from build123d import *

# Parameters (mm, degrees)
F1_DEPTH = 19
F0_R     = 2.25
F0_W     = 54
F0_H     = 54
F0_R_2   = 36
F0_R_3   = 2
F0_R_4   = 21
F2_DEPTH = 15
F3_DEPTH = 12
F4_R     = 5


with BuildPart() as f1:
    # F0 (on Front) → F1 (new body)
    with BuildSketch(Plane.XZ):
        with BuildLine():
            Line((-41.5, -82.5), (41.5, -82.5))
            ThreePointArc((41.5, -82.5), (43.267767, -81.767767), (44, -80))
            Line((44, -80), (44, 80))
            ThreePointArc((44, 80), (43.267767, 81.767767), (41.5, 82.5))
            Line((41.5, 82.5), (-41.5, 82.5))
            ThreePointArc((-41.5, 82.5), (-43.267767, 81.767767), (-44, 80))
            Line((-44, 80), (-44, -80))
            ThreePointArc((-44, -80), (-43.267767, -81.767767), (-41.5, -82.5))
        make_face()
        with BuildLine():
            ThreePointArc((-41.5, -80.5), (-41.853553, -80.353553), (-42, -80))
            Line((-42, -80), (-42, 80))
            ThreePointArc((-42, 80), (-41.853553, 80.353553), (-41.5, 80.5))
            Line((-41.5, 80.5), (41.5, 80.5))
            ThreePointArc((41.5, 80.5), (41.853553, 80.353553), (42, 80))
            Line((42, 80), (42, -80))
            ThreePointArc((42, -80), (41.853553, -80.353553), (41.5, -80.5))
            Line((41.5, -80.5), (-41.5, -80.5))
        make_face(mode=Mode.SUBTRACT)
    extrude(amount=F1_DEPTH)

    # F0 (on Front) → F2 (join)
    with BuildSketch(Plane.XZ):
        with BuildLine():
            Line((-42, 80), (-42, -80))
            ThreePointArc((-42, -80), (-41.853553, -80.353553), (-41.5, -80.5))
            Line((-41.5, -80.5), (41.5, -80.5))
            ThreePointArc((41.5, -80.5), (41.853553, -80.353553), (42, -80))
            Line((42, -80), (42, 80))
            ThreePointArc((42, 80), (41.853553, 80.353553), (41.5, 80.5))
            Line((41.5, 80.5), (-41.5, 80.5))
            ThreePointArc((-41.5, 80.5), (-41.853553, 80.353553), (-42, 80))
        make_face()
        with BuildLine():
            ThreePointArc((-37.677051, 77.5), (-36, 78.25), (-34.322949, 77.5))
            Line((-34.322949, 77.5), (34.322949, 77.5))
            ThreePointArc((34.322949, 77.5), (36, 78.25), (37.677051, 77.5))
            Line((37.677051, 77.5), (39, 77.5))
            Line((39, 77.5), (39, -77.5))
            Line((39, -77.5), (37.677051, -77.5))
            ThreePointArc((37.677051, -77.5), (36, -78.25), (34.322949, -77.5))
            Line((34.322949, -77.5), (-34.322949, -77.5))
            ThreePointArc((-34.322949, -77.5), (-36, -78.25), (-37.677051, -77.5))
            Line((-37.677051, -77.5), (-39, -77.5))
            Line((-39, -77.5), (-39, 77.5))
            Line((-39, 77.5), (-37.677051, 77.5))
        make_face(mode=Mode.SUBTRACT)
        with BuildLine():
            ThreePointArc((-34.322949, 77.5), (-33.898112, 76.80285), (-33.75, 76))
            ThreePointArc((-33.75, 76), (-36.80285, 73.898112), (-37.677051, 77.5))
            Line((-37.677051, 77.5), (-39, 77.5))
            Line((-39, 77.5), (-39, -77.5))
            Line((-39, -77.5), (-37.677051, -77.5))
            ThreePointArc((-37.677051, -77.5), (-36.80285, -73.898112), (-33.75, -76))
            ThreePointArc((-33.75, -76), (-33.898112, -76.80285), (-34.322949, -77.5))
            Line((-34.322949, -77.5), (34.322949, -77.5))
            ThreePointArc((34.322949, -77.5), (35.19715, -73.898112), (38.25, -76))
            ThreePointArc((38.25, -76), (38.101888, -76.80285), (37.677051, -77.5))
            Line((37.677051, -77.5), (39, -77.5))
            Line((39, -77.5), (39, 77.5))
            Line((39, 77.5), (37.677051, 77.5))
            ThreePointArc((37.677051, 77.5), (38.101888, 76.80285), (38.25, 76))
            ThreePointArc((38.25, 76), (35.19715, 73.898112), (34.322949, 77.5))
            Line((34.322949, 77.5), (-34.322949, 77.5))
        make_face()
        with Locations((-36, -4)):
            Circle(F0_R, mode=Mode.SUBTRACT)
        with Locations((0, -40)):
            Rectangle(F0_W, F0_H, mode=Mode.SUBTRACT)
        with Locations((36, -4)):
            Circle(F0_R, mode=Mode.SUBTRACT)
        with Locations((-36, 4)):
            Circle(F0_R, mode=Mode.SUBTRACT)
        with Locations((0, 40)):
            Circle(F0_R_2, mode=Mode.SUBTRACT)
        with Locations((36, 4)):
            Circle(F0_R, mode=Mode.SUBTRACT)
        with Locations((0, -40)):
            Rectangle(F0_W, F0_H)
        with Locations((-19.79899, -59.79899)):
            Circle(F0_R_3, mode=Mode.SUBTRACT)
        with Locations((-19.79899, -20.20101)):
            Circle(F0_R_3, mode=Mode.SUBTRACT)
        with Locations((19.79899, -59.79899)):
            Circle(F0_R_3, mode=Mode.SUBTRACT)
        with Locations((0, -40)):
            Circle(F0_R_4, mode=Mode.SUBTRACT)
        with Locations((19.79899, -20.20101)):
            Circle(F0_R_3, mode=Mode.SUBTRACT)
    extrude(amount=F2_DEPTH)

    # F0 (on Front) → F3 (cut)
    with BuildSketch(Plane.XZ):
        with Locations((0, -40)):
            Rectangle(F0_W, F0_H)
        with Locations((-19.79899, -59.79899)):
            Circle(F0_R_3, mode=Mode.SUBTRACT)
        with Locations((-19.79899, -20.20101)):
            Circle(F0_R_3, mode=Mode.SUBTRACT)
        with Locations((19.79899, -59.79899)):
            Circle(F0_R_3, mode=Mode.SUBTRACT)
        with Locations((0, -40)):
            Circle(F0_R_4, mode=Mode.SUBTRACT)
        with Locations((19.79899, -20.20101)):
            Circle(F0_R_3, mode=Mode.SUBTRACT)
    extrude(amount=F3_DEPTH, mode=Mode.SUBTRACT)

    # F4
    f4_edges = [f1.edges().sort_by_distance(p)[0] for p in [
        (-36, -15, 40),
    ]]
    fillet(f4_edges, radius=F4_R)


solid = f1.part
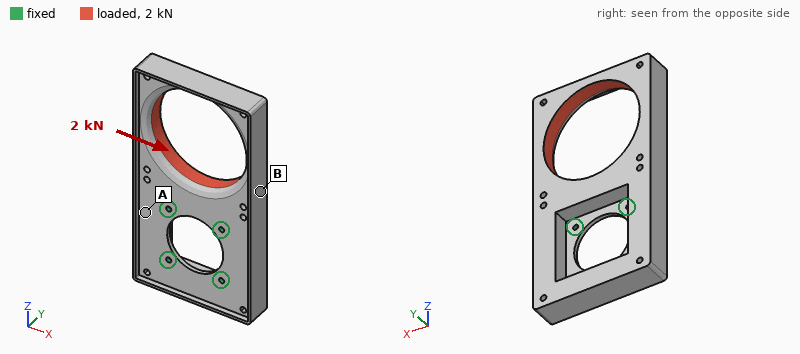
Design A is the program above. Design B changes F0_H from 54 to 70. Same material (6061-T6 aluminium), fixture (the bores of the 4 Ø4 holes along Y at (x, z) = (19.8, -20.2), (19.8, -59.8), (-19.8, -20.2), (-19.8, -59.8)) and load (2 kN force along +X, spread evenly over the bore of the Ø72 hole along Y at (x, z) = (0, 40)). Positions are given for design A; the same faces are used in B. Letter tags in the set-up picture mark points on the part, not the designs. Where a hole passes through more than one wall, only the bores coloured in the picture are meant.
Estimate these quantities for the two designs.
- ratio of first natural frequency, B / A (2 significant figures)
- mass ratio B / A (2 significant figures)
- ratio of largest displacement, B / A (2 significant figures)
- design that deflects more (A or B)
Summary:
0.95
0.91
1.2
B
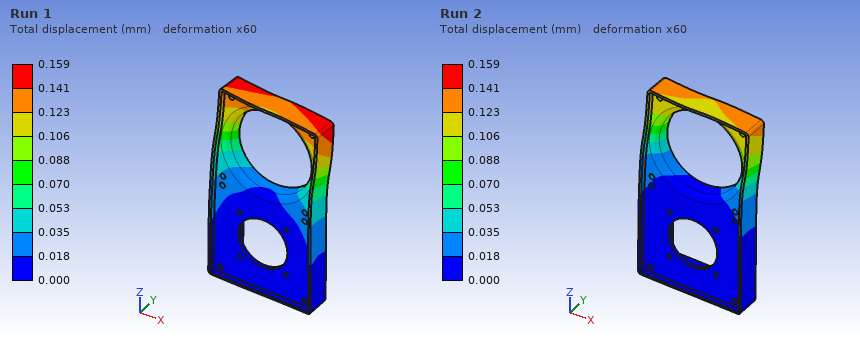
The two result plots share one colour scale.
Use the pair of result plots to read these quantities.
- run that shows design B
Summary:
Run 1
